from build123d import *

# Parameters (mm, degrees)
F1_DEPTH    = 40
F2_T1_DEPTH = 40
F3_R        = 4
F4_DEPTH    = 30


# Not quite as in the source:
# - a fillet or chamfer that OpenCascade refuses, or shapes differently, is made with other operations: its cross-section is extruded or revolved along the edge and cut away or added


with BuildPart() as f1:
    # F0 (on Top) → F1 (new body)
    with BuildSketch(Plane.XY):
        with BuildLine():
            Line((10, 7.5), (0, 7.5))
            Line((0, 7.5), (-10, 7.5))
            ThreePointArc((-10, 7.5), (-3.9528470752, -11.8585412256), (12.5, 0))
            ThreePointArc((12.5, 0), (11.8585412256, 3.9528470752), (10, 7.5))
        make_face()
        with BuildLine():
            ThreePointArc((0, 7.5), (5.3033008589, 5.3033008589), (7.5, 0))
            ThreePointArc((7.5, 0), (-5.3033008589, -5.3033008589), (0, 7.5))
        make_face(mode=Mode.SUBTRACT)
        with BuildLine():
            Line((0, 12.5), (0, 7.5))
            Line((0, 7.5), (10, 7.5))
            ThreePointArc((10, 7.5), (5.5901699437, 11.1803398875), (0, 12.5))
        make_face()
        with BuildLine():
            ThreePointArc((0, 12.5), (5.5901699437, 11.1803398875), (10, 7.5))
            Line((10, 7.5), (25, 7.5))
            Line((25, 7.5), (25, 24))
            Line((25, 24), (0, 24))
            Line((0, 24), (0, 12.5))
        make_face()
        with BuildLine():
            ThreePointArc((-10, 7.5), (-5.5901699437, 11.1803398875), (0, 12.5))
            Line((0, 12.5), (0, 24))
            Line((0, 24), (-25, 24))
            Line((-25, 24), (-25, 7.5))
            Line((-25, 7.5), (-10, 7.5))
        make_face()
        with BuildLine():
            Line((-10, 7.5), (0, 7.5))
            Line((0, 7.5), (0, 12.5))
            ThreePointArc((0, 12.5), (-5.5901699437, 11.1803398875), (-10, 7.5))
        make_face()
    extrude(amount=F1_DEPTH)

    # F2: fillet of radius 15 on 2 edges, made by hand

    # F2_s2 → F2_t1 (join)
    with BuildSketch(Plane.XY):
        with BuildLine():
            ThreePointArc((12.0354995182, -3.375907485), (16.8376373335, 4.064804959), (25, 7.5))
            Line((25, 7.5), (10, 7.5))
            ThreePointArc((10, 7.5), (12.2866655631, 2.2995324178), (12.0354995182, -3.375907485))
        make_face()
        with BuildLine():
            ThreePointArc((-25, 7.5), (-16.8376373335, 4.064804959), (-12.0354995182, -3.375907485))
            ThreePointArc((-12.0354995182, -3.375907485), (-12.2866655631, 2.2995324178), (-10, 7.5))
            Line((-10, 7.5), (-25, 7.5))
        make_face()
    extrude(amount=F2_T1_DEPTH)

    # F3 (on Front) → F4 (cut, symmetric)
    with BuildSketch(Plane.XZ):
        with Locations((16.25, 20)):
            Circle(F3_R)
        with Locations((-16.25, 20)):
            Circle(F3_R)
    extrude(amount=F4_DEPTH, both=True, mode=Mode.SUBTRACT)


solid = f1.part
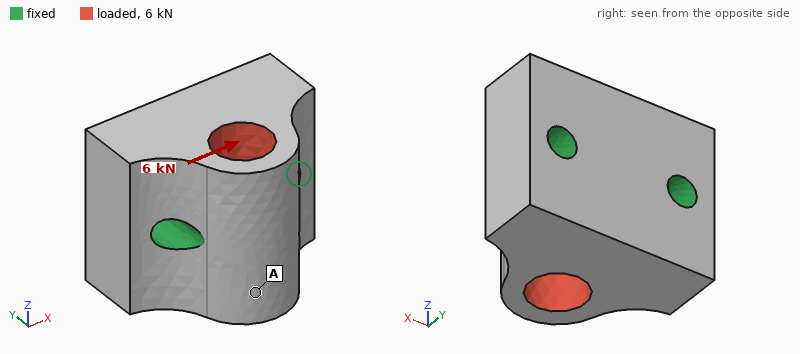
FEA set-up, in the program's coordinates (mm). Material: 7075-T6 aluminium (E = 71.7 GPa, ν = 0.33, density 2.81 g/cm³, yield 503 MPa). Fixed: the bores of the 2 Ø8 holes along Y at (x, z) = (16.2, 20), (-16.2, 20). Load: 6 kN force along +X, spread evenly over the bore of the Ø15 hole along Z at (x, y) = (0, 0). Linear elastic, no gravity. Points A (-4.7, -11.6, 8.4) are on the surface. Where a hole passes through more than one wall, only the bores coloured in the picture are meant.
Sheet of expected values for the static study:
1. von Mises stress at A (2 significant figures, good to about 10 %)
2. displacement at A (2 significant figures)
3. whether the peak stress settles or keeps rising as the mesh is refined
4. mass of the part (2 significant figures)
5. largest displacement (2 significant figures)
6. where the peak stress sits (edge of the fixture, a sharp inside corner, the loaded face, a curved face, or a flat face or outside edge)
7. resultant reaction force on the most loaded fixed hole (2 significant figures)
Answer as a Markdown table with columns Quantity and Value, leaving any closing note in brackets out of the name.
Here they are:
| Quantity | Value |
|---|---|
| von Mises stress at A | 7.8 MPa |
| displacement at A | 5.5 µm |
| whether the peak stress settles or keeps rising as the mesh is refined | keeps rising |
| mass of the part | 120 g |
| largest displacement | 6.7 µm |
| where the peak stress sits | edge of the fixture |
| resultant reaction force on the most loaded fixed hole | 3.3 kN |
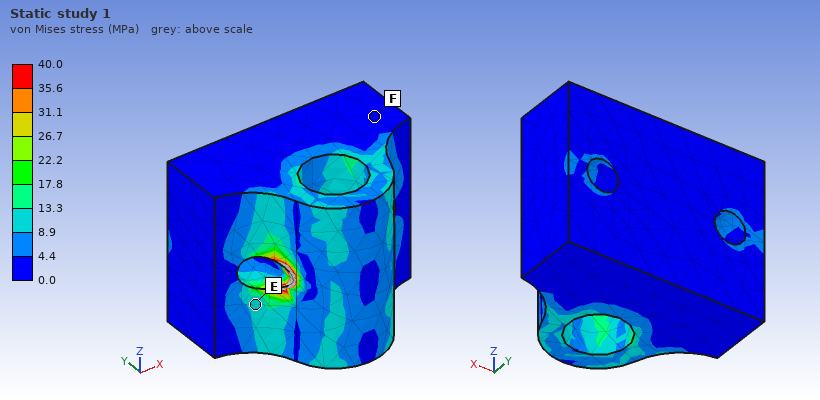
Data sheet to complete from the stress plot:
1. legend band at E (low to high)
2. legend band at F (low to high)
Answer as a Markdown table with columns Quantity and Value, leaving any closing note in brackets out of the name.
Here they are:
| Quantity | Value |
|---|---|
| legend band at E | 8.9 to 13.3 MPa |
| legend band at F | 0.0 to 4.4 MPa |
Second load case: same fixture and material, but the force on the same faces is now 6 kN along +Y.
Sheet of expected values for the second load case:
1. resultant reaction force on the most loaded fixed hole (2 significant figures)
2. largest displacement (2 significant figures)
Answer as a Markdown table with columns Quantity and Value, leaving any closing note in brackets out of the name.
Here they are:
| Quantity | Value |
|---|---|
| resultant reaction force on the most loaded fixed hole | 3.1 kN |
| largest displacement | 4.1 µm |
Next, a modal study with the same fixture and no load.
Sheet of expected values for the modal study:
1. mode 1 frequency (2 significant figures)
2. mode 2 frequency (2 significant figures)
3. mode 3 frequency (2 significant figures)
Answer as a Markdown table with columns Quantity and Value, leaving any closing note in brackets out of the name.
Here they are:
| Quantity | Value |
|---|---|
| mode 1 frequency | 22 kHz |
| mode 2 frequency | 28 kHz |
| mode 3 frequency | 29 kHz |
